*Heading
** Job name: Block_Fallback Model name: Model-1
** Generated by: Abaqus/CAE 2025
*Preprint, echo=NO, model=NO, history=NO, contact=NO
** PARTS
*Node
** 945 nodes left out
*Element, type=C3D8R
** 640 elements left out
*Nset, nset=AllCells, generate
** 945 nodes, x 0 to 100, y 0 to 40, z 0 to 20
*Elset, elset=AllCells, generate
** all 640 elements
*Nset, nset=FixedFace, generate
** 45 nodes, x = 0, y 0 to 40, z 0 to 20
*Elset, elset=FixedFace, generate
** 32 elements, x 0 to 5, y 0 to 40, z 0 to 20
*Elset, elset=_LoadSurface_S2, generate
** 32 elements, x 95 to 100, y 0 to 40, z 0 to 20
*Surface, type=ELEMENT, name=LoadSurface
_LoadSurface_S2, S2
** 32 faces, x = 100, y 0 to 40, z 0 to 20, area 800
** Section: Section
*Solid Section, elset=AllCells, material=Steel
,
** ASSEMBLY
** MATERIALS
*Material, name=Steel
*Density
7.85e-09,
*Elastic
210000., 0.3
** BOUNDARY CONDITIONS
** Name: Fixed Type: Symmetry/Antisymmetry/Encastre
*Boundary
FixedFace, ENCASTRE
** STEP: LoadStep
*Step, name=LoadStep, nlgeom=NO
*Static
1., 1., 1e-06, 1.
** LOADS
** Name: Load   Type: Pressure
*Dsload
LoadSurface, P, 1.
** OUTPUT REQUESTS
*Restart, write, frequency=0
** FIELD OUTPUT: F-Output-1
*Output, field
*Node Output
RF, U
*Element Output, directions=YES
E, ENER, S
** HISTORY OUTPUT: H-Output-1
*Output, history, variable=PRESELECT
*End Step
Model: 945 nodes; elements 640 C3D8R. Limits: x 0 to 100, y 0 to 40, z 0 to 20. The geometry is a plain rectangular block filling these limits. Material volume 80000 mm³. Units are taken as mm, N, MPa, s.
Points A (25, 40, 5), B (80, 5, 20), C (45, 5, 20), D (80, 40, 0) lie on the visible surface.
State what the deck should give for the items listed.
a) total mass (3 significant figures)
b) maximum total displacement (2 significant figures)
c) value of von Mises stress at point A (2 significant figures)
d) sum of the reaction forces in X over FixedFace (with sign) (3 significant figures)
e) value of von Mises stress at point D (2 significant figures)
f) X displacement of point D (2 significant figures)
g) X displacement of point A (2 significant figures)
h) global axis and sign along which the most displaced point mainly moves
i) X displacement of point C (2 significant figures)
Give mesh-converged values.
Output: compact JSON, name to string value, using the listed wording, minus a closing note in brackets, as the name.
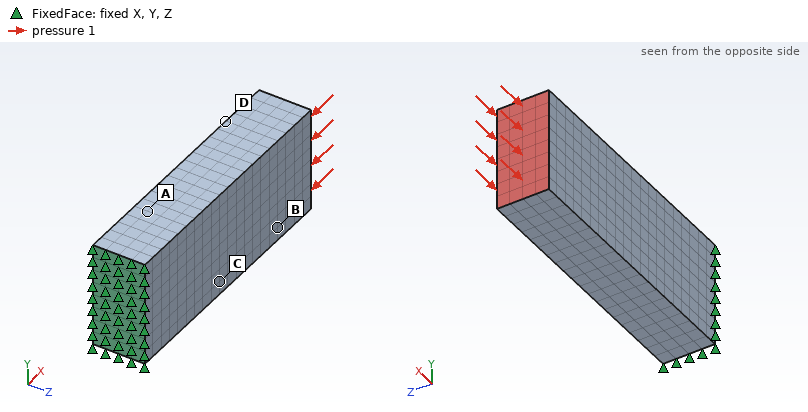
{"total mass": "0.628 kg", "maximum total displacement": "4.7e-04 mm", "value of von Mises stress at point A": "0.97 MPa", "sum of the reaction forces in X over FixedFace (with sign)": "800 N", "value of von Mises stress at point D": "1.0 MPa", "X displacement of point D": "-3.8e-04 mm", "X displacement of point A": "-1.2e-04 mm", "global axis and sign along which the most displaced point mainly moves": "-X", "X displacement of point C": "-2.1e-04 mm"}
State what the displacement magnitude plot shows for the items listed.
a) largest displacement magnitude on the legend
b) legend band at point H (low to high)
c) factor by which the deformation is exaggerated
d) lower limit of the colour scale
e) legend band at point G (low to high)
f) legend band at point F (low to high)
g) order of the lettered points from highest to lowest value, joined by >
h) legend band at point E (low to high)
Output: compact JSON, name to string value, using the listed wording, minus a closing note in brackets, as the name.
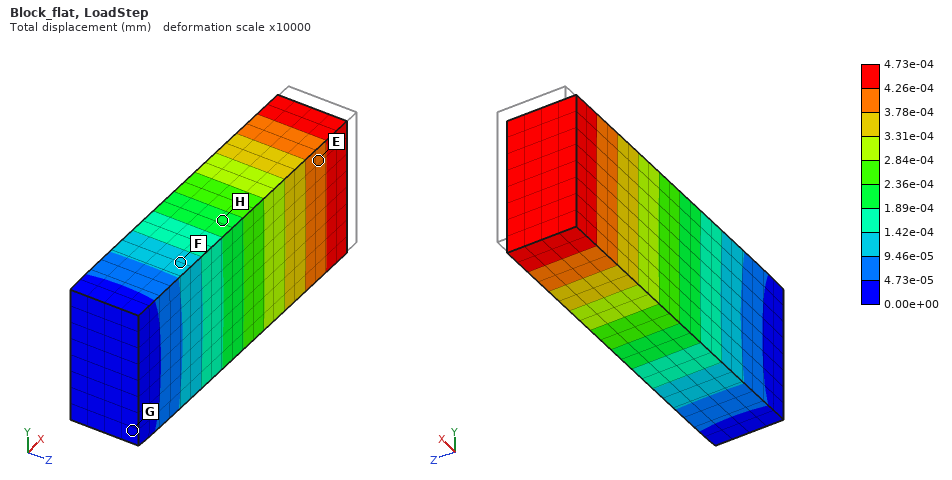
{"largest displacement magnitude on the legend": "4.73e-04 mm", "legend band at point H": "1.89e-04 to 2.36e-04 mm", "factor by which the deformation is exaggerated": "10000", "lower limit of the colour scale": "0.00e+00 mm", "legend band at point G": "0.00e+00 to 4.73e-05 mm", "legend band at point F": "9.46e-05 to 1.42e-04 mm", "order of the lettered points from highest to lowest value, joined by >": "E > H > F > G", "legend band at point E": "3.78e-04 to 4.26e-04 mm"}
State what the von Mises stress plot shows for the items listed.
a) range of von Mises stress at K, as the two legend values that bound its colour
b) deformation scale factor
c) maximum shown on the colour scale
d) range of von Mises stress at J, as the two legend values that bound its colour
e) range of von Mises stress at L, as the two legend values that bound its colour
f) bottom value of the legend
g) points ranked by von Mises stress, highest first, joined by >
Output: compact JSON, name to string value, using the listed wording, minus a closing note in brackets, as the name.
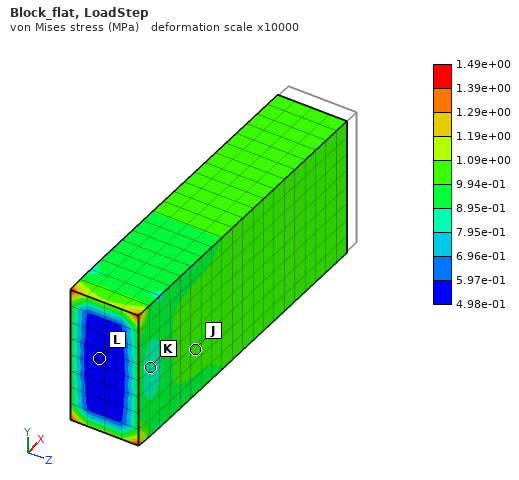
{"range of von Mises stress at K, as the two legend values that bound its colour": "7.95e-01 to 8.95e-01 MPa", "deformation scale factor": "10000", "maximum shown on the colour scale": "1.49e+00 MPa", "range of von Mises stress at J, as the two legend values that bound its colour": "9.94e-01 to 1.09e+00 MPa", "range of von Mises stress at L, as the two legend values that bound its colour": "4.98e-01 to 5.97e-01 MPa", "bottom value of the legend": "4.98e-01 MPa", "points ranked by von Mises stress, highest first, joined by >": "J > K > L"}
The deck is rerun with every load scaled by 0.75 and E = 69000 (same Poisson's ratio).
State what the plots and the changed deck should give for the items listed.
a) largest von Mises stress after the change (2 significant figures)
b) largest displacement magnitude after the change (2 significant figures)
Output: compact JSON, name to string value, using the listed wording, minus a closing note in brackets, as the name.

{"largest von Mises stress after the change": "1.1 MPa", "largest displacement magnitude after the change": "0.0011 mm"}
